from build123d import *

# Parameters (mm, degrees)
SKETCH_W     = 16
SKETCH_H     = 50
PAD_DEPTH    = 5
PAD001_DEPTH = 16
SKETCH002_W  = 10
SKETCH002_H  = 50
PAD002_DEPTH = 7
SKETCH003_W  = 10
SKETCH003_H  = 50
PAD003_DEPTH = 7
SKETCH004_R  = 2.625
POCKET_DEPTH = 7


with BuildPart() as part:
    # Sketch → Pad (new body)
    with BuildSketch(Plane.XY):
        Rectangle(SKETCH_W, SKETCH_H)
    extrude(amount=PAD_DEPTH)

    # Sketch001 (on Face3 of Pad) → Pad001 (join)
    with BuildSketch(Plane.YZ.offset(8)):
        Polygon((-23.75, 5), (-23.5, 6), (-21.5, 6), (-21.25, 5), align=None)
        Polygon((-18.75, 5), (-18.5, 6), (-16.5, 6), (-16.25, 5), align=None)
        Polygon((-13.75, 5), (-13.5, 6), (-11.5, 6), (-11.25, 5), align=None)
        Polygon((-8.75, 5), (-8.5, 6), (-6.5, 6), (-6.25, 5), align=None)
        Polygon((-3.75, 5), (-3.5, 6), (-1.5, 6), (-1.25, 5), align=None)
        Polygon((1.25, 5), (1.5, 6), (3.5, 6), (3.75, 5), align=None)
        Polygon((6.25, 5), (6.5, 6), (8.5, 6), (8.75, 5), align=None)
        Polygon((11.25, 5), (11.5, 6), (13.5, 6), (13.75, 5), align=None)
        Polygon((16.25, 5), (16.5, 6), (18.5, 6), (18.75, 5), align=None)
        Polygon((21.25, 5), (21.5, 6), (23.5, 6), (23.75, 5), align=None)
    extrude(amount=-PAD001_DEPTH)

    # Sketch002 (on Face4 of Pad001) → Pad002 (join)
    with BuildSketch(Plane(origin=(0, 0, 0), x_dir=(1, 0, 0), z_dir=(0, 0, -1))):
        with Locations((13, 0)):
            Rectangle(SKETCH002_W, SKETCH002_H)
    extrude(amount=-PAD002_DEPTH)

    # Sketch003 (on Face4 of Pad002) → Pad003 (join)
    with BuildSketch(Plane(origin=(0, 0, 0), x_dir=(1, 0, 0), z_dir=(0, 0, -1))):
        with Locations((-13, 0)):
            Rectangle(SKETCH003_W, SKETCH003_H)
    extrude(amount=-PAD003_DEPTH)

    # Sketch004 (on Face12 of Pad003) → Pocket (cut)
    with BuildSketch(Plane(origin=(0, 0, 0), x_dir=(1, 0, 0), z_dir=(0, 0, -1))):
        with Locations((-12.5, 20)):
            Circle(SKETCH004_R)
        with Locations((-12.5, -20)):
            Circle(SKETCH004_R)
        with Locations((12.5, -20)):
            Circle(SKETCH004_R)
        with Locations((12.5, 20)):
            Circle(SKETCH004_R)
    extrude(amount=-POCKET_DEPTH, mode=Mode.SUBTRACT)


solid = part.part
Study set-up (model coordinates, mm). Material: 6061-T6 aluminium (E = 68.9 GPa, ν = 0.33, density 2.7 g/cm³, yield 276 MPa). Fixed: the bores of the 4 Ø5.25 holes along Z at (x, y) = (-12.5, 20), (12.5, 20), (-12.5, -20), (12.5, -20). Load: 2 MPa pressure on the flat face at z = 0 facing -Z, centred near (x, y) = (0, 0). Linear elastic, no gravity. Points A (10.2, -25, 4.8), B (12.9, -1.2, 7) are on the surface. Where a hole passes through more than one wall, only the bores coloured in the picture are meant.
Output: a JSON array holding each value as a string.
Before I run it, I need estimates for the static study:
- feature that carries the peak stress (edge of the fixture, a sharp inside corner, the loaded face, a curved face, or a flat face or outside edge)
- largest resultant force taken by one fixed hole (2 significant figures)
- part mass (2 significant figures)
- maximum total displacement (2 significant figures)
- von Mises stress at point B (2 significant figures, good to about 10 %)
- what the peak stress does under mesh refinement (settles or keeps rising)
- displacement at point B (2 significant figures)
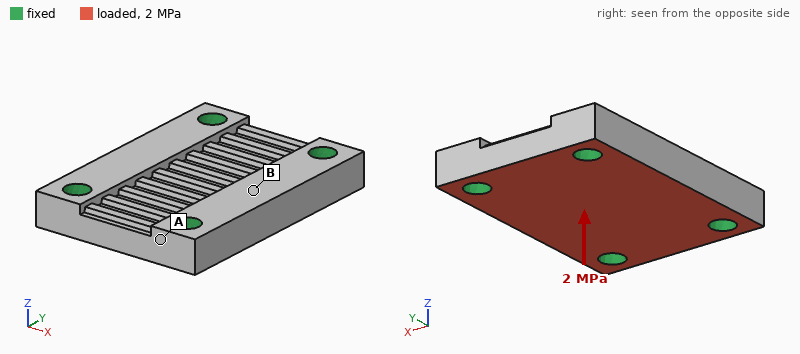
["edge of the fixture", "870 N", "29 g", "12 µm", "19 MPa", "keeps rising", "9.4 µm"]
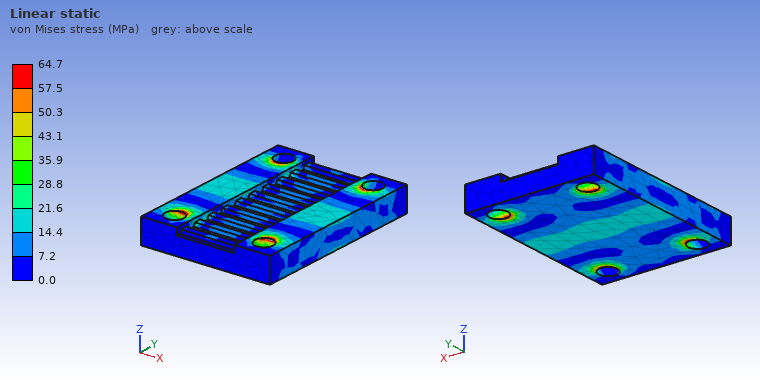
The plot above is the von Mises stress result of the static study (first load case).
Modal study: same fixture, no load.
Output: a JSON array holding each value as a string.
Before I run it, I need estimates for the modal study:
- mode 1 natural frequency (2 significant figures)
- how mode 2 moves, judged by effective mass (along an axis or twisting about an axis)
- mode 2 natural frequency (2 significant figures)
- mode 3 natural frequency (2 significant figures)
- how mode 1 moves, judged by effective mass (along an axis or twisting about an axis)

["19 kHz", "twisting about Y", "24 kHz", "33 kHz", "along Z"]
